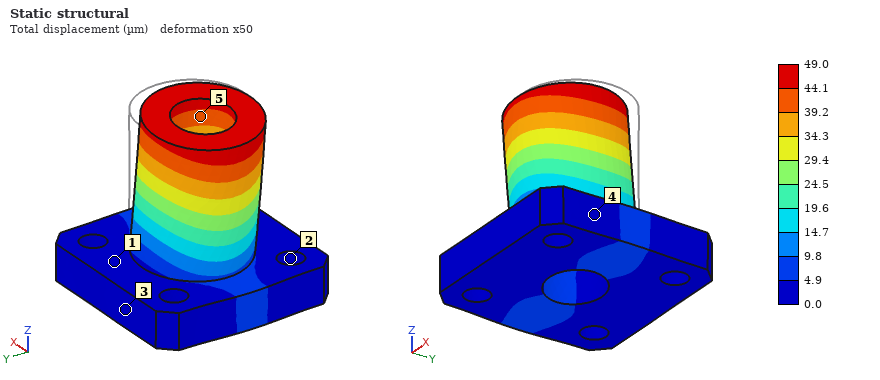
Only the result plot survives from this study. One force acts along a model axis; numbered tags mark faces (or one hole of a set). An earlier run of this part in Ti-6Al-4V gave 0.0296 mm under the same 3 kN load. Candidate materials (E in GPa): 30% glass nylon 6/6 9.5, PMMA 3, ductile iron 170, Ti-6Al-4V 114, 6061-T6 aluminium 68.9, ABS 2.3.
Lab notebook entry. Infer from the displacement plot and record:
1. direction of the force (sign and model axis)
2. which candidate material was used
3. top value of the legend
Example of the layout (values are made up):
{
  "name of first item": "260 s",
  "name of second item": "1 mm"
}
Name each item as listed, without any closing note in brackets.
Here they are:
{
  "direction of the force": "-X",
  "which candidate material was used": "6061-T6 aluminium",
  "top value of the legend": "49.0 µm"
}
